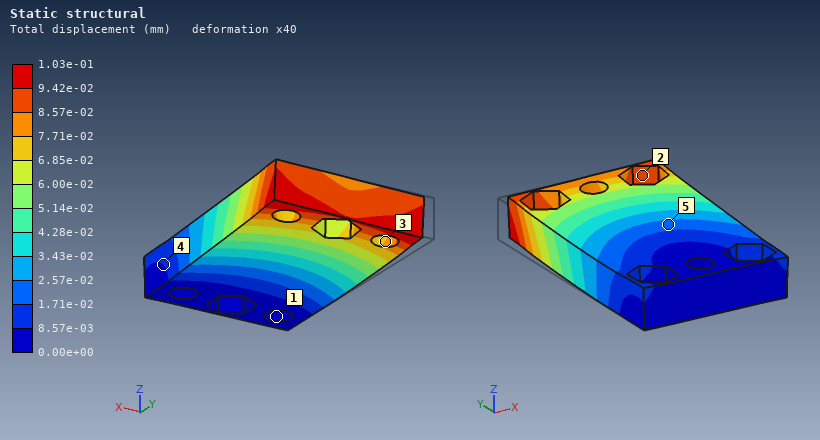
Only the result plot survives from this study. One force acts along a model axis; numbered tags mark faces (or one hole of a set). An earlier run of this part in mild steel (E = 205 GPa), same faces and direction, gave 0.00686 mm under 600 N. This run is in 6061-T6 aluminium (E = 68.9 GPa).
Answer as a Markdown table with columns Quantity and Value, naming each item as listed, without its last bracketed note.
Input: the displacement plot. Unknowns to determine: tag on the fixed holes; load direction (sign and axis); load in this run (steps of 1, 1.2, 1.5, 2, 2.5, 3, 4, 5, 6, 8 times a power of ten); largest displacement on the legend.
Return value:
| Quantity | Value |
|---|---|
| tag on the fixed holes | 1 |
| load direction | +X |
| load in this run | 3 kN |
| largest displacement on the legend | 1.03e-01 mm |
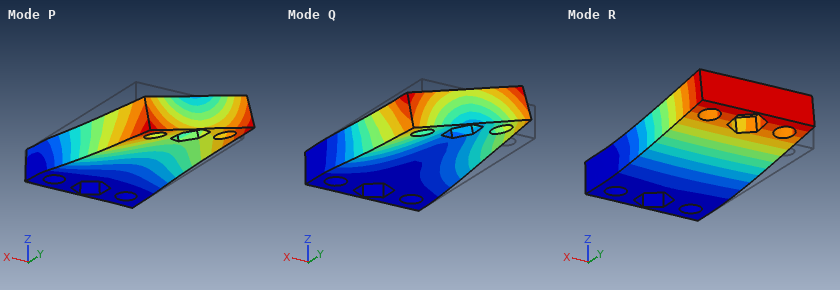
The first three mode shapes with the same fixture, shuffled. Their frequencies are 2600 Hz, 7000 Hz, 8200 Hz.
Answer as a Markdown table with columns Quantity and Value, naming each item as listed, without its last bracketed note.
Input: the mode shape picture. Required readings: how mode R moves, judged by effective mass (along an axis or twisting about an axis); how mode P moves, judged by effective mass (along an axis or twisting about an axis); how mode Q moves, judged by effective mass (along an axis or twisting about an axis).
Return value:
| Quantity | Value |
|---|---|
| how mode R moves, judged by effective mass | along Z |
| how mode P moves, judged by effective mass | along X |
| how mode Q moves, judged by effective mass | along X |
